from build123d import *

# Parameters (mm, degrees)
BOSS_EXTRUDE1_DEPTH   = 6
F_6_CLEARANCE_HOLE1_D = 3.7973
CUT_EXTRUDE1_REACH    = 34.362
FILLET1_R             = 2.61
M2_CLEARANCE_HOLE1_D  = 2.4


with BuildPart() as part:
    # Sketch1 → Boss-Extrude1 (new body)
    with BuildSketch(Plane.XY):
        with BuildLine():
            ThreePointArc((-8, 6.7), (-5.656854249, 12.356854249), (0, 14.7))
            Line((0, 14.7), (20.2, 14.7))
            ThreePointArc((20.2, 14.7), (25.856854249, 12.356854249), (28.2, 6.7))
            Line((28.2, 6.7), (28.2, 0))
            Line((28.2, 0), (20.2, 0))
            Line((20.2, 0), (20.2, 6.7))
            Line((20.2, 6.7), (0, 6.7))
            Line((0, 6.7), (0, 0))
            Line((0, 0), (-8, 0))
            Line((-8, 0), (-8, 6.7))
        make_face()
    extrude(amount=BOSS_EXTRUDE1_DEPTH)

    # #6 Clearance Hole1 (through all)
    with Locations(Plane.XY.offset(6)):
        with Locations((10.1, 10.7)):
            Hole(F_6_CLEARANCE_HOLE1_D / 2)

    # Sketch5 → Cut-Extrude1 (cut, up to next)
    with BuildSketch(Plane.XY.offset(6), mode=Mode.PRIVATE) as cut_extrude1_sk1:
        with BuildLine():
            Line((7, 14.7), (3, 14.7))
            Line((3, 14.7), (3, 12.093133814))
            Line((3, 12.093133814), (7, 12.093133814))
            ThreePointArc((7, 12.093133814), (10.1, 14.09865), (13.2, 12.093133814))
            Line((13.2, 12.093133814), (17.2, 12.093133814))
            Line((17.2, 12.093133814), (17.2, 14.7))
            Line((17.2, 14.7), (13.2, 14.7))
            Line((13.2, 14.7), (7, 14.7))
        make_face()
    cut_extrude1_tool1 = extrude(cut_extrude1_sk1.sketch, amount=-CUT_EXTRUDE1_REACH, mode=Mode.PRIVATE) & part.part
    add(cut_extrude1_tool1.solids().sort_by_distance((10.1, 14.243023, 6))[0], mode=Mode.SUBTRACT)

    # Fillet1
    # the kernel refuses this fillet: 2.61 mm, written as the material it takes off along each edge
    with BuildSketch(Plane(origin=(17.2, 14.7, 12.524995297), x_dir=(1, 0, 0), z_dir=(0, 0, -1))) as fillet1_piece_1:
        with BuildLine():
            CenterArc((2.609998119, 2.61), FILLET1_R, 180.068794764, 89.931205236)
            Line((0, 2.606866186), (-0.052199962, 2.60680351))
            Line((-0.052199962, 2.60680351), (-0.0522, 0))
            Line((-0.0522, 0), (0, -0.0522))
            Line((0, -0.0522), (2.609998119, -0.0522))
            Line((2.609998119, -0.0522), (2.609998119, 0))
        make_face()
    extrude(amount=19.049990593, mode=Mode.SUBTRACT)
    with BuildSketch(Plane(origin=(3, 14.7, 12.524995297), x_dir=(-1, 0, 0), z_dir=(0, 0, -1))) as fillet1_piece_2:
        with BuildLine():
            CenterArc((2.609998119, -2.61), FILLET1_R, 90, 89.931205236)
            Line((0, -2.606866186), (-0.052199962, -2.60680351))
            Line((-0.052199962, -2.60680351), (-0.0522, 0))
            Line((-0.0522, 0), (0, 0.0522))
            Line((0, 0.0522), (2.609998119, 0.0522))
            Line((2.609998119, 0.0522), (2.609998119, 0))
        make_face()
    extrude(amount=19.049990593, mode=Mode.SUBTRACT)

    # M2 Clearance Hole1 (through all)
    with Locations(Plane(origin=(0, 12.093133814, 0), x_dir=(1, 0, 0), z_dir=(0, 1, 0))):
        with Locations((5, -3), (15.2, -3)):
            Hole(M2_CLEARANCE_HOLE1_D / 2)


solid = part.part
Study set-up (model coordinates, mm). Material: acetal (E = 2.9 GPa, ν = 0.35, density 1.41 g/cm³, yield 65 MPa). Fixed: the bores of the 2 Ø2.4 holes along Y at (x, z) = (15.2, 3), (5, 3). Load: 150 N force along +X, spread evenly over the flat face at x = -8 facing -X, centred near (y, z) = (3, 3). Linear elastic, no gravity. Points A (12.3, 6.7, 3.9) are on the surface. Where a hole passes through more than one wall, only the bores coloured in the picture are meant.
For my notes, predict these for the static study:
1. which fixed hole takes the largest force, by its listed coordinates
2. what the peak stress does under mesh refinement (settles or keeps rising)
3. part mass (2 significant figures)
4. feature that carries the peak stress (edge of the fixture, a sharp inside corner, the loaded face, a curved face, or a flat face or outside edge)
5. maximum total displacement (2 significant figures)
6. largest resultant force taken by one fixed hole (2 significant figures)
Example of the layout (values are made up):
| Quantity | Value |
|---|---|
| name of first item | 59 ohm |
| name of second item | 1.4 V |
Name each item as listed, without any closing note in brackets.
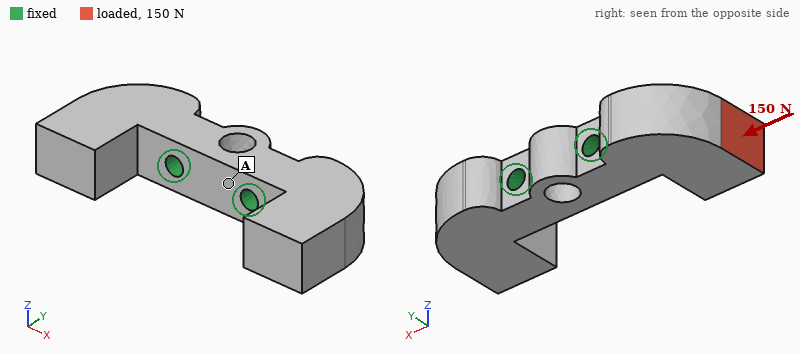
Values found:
| Quantity | Value |
|---|---|
| which fixed hole takes the largest force, by its listed coordinates | (5, 3) |
| what the peak stress does under mesh refinement | keeps rising |
| part mass | 2.7 g |
| feature that carries the peak stress | edge of the fixture |
| maximum total displacement | 0.32 mm |
| largest resultant force taken by one fixed hole | 140 N |
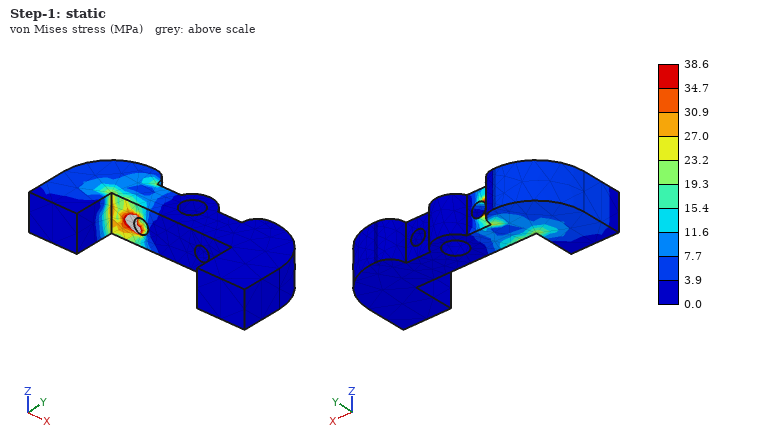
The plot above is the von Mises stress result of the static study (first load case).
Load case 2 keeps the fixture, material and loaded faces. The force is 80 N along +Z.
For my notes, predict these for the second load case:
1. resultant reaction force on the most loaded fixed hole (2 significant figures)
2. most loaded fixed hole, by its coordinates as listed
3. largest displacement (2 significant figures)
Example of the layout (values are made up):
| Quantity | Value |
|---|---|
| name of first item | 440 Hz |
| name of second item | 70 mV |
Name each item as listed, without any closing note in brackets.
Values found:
| Quantity | Value |
|---|---|
| resultant reaction force on the most loaded fixed hole | 110 N |
| most loaded fixed hole, by its coordinates as listed | (5, 3) |
| largest displacement | 0.46 mm |
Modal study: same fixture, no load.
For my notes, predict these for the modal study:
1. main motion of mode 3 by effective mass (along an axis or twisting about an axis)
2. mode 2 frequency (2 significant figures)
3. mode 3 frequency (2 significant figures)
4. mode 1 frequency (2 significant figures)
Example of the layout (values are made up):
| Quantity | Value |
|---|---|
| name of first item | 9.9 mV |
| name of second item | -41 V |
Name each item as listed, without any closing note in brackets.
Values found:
| Quantity | Value |
|---|---|
| main motion of mode 3 by effective mass | along Y |
| mode 2 frequency | 3900 Hz |
| mode 3 frequency | 4300 Hz |
| mode 1 frequency | 3900 Hz |
